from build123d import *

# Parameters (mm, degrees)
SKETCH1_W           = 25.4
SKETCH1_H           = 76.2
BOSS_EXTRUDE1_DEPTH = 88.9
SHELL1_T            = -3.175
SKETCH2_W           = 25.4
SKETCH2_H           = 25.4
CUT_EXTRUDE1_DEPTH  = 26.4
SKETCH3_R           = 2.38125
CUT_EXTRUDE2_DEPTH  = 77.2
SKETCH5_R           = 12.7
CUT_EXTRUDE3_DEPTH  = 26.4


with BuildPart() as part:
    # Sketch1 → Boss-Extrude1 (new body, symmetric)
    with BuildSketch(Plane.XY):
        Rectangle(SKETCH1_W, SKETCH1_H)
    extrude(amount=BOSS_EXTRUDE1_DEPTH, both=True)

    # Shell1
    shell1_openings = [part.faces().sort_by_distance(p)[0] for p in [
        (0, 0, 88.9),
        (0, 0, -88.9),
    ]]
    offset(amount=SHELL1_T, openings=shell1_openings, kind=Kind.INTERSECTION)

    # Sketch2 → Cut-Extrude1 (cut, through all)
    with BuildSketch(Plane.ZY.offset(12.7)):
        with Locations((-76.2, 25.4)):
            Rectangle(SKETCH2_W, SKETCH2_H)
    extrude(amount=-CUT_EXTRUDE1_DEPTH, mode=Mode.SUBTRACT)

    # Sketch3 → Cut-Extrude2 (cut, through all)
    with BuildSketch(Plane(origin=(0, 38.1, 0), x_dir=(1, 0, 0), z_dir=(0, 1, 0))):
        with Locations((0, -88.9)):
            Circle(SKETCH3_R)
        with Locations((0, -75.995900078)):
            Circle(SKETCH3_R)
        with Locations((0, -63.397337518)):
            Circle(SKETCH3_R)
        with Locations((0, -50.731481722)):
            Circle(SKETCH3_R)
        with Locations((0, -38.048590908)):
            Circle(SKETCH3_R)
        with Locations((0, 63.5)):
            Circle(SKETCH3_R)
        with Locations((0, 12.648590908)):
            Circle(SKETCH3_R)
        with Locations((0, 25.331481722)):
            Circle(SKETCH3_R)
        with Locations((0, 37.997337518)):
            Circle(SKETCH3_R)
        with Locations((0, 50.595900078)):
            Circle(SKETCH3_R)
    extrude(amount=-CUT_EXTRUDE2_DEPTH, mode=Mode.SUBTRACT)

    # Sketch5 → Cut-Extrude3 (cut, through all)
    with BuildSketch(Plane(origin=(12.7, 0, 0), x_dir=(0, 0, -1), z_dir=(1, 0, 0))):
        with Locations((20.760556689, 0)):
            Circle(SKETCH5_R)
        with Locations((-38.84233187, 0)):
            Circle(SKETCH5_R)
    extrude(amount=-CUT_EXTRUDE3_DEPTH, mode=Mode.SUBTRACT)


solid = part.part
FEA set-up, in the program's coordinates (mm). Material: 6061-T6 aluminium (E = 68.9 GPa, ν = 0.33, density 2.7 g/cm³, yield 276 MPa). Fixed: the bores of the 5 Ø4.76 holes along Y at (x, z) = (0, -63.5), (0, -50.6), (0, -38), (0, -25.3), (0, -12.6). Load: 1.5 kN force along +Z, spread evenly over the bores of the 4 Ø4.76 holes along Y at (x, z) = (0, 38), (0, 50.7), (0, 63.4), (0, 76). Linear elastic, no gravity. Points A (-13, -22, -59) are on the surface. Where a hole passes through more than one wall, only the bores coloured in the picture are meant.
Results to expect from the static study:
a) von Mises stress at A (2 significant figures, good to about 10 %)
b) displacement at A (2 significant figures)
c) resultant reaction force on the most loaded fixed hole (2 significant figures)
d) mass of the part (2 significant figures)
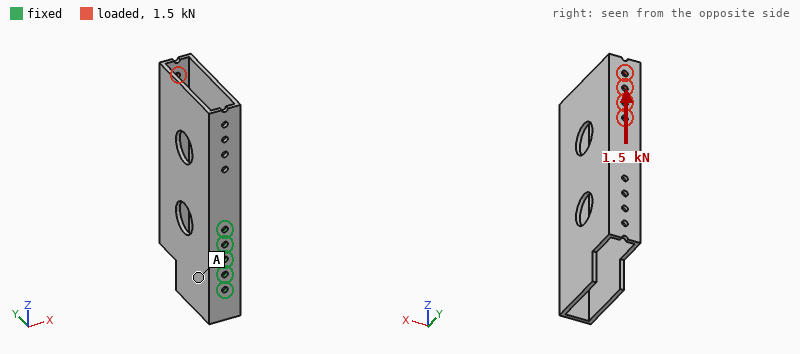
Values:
13 MPa
0.056 mm
1.8 kN
250 g
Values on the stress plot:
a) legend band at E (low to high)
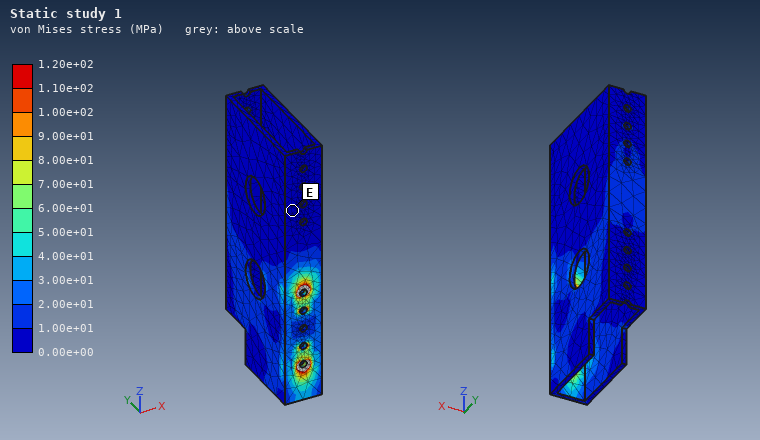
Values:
0.00e+00 to 1.00e+01 MPa
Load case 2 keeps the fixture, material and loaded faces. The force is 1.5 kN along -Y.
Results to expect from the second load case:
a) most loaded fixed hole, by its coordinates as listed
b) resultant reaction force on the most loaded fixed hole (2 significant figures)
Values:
(0, -12.6)
2.8 kN
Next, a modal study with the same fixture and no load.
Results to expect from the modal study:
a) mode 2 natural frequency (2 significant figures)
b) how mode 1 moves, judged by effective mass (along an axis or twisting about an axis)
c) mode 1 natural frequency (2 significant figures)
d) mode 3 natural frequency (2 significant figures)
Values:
910 Hz
along X
410 Hz
980 Hz
